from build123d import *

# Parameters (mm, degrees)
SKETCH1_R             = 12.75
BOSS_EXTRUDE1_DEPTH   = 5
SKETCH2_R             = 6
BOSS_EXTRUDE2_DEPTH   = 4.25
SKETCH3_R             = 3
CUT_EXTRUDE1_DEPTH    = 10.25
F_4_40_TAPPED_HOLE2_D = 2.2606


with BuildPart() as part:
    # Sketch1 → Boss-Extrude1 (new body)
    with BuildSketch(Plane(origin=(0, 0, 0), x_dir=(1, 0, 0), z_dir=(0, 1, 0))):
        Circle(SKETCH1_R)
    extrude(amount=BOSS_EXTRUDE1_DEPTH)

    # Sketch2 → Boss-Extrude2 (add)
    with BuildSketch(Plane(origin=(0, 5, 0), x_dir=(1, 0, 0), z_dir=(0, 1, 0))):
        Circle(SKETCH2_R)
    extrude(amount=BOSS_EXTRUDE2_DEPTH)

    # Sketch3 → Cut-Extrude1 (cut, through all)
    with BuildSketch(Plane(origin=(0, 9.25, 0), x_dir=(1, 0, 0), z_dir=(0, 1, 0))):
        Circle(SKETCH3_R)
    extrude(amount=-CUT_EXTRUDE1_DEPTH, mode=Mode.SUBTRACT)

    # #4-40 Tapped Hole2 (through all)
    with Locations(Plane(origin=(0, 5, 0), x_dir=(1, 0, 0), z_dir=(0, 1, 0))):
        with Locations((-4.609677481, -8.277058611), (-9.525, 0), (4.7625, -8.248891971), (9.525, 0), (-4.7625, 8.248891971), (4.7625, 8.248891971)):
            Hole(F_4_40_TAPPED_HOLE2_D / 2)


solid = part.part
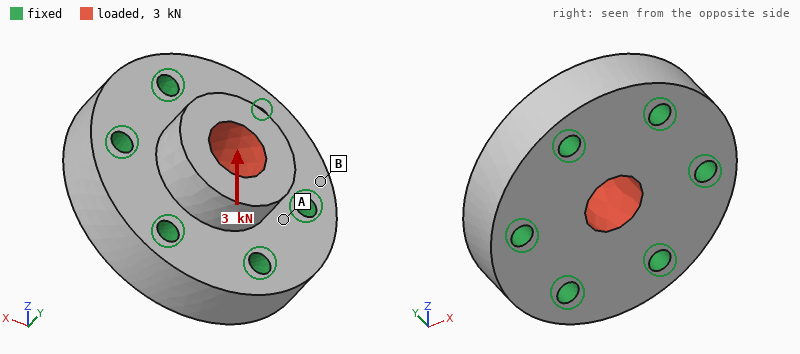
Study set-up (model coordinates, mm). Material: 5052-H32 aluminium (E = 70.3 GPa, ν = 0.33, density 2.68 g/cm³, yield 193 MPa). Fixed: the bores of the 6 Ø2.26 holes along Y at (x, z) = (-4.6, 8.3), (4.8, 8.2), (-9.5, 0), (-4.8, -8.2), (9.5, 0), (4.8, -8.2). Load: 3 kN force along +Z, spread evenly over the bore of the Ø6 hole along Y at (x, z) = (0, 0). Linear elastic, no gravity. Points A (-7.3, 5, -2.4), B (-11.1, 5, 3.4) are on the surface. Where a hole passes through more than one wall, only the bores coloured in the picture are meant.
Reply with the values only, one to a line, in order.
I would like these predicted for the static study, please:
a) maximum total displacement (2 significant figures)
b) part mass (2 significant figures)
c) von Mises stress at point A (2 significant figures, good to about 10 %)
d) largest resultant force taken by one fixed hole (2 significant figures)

6.6 µm
7.1 g
12 MPa
710 N
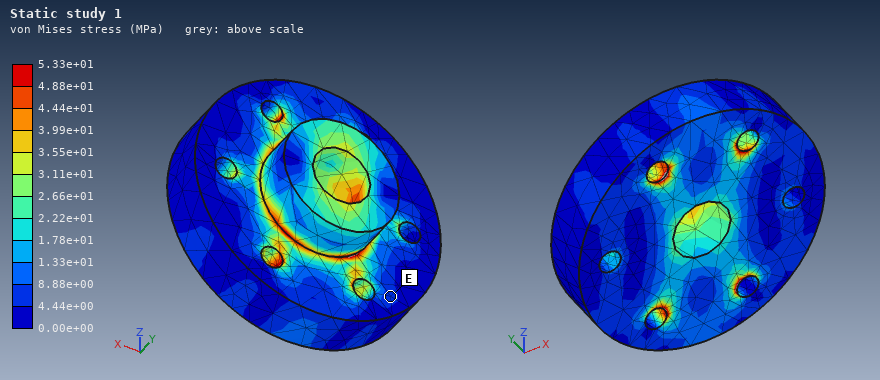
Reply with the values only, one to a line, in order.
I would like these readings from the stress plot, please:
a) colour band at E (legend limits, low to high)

4.44e+00 to 8.88e+00 MPa
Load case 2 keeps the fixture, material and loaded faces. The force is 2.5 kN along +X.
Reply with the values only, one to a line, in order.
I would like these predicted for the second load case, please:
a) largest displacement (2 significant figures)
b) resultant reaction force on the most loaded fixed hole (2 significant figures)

5.5 µm
660 N
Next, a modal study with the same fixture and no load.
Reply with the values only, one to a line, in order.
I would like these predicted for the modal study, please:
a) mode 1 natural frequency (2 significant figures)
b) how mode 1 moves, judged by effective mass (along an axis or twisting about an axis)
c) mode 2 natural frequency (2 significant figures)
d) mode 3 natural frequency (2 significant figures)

84 kHz
along Y
90 kHz
91 kHz
